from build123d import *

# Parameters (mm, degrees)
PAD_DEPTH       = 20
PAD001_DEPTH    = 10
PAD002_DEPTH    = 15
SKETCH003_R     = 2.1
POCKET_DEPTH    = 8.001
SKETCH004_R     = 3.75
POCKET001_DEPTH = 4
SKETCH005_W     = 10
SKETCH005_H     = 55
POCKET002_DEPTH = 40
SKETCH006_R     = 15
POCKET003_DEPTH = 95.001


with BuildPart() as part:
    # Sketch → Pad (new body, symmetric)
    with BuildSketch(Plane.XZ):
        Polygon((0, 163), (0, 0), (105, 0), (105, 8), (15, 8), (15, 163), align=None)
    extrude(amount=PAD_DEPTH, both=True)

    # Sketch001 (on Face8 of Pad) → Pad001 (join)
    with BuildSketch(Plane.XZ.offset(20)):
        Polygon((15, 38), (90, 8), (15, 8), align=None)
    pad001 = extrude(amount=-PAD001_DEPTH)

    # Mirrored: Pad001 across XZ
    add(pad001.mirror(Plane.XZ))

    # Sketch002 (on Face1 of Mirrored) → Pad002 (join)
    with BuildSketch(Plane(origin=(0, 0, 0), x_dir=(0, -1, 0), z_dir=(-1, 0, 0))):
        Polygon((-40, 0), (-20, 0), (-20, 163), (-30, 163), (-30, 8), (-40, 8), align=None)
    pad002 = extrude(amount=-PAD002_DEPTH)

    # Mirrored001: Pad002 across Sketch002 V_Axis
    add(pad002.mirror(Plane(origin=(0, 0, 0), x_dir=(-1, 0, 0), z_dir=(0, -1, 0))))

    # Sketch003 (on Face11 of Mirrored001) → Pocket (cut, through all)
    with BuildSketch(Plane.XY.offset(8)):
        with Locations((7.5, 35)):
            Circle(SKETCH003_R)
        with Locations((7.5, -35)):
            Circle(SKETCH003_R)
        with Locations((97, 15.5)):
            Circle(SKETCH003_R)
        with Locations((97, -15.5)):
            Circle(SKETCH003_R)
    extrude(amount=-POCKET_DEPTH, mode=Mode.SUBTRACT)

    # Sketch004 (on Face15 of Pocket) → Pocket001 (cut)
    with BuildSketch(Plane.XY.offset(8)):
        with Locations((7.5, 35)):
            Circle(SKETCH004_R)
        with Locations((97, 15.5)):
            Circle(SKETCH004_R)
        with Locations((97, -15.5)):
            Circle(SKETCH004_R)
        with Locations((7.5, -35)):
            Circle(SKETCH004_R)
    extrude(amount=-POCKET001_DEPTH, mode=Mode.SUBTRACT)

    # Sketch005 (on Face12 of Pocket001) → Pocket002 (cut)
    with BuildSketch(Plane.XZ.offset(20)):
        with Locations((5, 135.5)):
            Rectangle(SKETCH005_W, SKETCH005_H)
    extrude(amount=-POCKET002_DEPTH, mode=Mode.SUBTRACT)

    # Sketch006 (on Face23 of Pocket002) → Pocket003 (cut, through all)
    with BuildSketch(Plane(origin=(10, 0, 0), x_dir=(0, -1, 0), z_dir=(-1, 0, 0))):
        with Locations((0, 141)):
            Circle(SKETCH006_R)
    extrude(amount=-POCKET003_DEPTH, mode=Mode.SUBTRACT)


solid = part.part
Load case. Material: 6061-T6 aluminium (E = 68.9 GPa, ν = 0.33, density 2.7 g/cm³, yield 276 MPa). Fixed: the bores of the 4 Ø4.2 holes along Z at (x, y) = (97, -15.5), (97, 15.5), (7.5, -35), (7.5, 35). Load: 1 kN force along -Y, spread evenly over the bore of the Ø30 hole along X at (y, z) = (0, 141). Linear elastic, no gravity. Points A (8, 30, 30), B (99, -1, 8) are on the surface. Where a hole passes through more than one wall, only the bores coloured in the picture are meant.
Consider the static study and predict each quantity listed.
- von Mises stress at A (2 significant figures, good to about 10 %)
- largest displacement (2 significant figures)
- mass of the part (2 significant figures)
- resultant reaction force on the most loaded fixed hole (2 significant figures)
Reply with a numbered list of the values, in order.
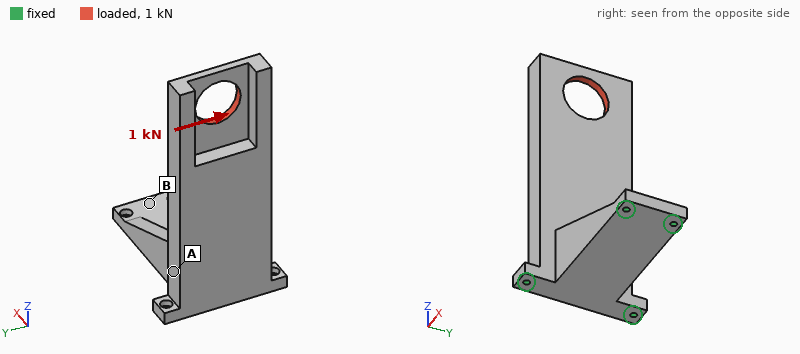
1. 13 MPa
2. 0.15 mm
3. 470 g
4. 2.1 kN
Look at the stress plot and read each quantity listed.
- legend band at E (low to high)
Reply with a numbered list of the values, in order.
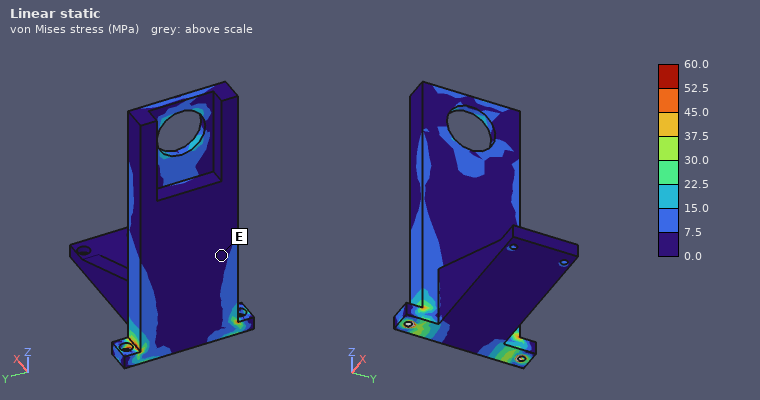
1. 0.0 to 7.5 MPa
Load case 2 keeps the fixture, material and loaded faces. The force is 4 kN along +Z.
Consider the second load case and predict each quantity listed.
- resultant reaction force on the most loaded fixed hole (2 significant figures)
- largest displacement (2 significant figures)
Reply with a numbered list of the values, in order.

1. 2.2 kN
2. 0.16 mm
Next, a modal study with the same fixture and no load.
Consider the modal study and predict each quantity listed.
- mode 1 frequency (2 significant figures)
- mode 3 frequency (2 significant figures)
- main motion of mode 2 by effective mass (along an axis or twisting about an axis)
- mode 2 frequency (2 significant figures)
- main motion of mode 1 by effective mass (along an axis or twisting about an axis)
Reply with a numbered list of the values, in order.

1. 750 Hz
2. 2200 Hz
3. along Y
4. 1500 Hz
5. along X
